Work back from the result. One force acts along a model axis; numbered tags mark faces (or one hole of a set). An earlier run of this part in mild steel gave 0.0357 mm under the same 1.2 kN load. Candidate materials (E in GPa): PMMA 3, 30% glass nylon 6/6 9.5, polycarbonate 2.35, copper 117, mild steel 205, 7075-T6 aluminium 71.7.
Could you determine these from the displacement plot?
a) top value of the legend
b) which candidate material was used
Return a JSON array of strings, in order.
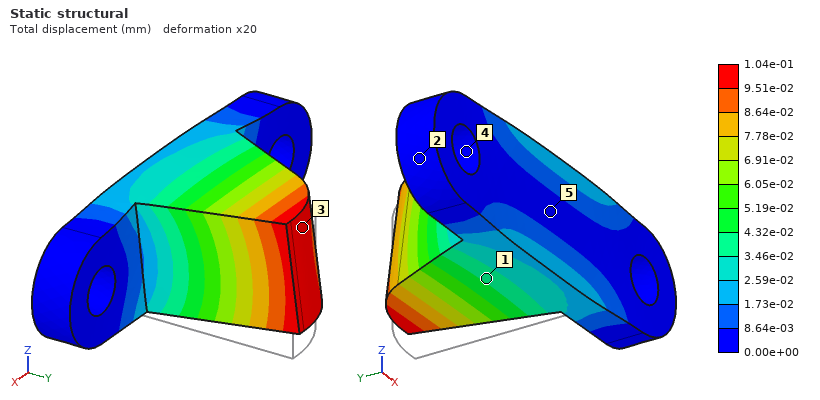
["1.04e-01 mm", "7075-T6 aluminium"]
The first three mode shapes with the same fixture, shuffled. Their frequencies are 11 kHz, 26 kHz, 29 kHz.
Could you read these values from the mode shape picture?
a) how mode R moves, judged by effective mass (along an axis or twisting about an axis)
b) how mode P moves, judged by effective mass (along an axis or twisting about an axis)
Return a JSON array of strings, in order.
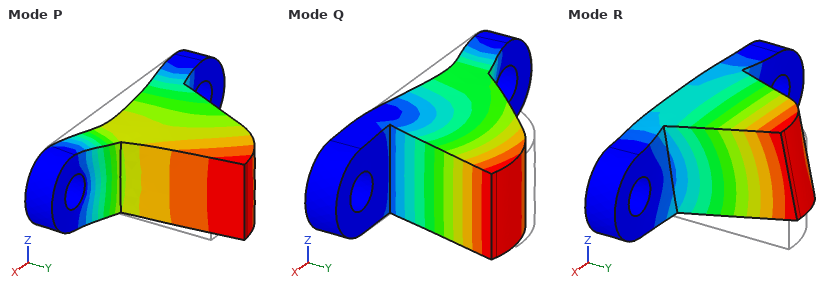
["along Z", "along Y"]
